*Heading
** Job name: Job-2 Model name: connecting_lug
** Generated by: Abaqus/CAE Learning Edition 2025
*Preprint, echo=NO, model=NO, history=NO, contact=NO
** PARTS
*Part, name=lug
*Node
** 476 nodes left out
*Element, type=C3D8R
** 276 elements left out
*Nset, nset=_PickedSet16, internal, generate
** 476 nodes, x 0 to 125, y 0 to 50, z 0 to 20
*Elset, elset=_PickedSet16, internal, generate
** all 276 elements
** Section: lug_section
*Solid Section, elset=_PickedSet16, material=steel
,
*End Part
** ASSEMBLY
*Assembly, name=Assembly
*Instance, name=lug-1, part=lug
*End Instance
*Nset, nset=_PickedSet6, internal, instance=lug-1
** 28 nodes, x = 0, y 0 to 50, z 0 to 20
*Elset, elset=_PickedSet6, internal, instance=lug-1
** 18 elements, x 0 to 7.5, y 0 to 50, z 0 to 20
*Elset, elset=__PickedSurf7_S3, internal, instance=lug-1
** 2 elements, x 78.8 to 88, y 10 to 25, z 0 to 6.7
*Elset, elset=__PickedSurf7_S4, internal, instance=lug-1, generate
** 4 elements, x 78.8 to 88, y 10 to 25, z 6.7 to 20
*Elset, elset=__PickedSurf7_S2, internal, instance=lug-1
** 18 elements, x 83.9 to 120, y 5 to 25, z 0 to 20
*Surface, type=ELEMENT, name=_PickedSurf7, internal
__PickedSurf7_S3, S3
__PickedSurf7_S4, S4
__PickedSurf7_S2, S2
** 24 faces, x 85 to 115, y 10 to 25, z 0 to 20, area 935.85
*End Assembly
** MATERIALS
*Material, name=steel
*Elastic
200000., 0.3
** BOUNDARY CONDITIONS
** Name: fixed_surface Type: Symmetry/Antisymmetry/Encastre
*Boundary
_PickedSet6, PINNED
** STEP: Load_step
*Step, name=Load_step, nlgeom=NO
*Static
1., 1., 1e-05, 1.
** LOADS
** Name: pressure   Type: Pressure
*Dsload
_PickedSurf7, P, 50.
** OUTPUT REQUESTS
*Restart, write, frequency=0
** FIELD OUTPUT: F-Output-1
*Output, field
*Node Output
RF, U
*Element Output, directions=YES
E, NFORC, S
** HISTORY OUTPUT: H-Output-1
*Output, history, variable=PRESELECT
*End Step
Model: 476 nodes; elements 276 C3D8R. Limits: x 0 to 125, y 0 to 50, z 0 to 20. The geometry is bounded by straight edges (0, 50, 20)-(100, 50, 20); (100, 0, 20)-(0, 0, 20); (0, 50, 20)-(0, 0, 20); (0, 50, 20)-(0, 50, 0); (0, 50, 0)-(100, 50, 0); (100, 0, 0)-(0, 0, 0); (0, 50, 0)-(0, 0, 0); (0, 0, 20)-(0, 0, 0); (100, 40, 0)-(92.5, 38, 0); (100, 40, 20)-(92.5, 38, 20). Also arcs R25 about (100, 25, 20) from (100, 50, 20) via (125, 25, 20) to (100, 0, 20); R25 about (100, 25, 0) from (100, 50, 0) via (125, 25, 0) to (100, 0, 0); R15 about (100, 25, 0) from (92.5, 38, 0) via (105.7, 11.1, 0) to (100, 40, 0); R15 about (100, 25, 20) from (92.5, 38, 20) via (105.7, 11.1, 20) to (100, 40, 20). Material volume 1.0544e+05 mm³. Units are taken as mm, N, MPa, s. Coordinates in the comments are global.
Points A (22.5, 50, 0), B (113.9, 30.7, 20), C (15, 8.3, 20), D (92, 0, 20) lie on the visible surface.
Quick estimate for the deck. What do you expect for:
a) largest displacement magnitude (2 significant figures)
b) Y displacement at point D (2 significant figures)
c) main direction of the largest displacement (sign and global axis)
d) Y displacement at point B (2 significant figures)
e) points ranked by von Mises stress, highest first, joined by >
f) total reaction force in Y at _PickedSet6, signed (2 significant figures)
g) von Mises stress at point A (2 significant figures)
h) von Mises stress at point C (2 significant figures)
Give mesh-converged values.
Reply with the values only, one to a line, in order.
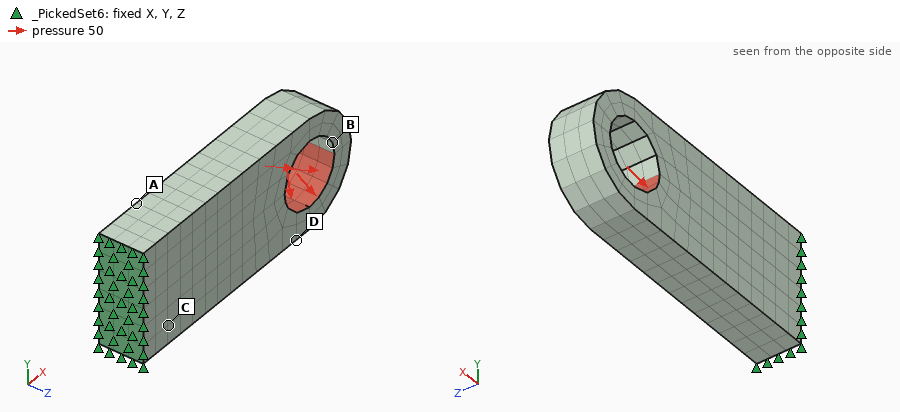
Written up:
0.42 mm
-0.26 mm
-Y
-0.39 mm
A > B > C > D
30000 N
280 MPa
210 MPa
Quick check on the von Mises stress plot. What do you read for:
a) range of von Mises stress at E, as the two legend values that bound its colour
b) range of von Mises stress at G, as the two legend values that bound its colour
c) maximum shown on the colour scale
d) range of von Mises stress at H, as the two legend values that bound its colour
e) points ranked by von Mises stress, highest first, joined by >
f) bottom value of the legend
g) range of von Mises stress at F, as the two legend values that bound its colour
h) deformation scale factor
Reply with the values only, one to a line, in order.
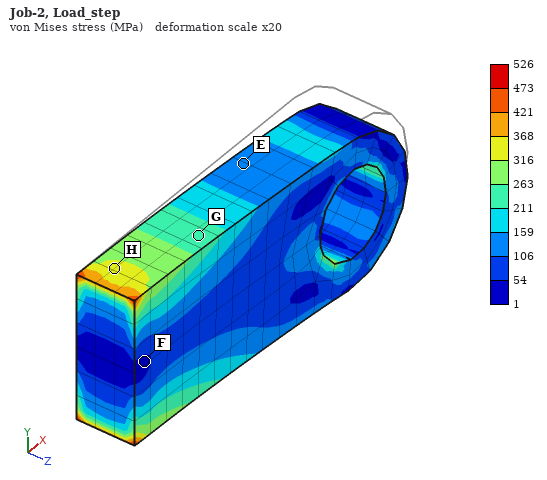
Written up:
106 to 159 MPa
211 to 263 MPa
526 MPa
316 to 368 MPa
H > G > E > F
1 MPa
1 to 54 MPa
20
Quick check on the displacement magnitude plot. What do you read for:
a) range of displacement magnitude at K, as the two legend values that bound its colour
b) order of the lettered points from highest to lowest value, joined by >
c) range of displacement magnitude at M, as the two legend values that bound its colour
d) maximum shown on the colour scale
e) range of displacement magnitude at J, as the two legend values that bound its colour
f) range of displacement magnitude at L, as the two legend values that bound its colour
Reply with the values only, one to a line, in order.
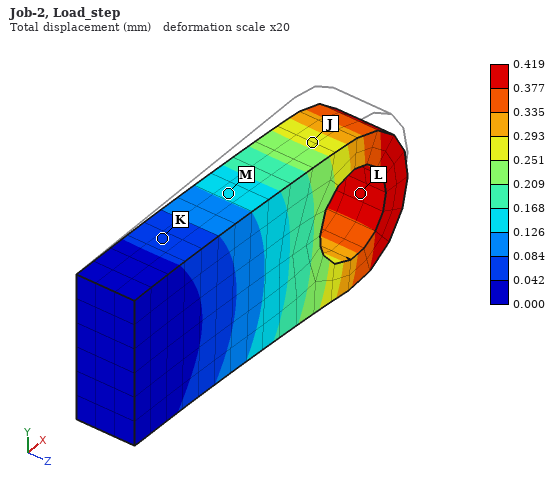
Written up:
0.042 to 0.084 mm
L > J > M > K
0.126 to 0.168 mm
0.419 mm
0.251 to 0.293 mm
0.377 to 0.419 mm
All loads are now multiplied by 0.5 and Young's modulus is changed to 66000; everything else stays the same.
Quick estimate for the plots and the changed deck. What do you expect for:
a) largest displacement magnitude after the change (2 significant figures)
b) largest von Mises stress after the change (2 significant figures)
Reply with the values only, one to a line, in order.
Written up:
0.63 mm
260 MPa
